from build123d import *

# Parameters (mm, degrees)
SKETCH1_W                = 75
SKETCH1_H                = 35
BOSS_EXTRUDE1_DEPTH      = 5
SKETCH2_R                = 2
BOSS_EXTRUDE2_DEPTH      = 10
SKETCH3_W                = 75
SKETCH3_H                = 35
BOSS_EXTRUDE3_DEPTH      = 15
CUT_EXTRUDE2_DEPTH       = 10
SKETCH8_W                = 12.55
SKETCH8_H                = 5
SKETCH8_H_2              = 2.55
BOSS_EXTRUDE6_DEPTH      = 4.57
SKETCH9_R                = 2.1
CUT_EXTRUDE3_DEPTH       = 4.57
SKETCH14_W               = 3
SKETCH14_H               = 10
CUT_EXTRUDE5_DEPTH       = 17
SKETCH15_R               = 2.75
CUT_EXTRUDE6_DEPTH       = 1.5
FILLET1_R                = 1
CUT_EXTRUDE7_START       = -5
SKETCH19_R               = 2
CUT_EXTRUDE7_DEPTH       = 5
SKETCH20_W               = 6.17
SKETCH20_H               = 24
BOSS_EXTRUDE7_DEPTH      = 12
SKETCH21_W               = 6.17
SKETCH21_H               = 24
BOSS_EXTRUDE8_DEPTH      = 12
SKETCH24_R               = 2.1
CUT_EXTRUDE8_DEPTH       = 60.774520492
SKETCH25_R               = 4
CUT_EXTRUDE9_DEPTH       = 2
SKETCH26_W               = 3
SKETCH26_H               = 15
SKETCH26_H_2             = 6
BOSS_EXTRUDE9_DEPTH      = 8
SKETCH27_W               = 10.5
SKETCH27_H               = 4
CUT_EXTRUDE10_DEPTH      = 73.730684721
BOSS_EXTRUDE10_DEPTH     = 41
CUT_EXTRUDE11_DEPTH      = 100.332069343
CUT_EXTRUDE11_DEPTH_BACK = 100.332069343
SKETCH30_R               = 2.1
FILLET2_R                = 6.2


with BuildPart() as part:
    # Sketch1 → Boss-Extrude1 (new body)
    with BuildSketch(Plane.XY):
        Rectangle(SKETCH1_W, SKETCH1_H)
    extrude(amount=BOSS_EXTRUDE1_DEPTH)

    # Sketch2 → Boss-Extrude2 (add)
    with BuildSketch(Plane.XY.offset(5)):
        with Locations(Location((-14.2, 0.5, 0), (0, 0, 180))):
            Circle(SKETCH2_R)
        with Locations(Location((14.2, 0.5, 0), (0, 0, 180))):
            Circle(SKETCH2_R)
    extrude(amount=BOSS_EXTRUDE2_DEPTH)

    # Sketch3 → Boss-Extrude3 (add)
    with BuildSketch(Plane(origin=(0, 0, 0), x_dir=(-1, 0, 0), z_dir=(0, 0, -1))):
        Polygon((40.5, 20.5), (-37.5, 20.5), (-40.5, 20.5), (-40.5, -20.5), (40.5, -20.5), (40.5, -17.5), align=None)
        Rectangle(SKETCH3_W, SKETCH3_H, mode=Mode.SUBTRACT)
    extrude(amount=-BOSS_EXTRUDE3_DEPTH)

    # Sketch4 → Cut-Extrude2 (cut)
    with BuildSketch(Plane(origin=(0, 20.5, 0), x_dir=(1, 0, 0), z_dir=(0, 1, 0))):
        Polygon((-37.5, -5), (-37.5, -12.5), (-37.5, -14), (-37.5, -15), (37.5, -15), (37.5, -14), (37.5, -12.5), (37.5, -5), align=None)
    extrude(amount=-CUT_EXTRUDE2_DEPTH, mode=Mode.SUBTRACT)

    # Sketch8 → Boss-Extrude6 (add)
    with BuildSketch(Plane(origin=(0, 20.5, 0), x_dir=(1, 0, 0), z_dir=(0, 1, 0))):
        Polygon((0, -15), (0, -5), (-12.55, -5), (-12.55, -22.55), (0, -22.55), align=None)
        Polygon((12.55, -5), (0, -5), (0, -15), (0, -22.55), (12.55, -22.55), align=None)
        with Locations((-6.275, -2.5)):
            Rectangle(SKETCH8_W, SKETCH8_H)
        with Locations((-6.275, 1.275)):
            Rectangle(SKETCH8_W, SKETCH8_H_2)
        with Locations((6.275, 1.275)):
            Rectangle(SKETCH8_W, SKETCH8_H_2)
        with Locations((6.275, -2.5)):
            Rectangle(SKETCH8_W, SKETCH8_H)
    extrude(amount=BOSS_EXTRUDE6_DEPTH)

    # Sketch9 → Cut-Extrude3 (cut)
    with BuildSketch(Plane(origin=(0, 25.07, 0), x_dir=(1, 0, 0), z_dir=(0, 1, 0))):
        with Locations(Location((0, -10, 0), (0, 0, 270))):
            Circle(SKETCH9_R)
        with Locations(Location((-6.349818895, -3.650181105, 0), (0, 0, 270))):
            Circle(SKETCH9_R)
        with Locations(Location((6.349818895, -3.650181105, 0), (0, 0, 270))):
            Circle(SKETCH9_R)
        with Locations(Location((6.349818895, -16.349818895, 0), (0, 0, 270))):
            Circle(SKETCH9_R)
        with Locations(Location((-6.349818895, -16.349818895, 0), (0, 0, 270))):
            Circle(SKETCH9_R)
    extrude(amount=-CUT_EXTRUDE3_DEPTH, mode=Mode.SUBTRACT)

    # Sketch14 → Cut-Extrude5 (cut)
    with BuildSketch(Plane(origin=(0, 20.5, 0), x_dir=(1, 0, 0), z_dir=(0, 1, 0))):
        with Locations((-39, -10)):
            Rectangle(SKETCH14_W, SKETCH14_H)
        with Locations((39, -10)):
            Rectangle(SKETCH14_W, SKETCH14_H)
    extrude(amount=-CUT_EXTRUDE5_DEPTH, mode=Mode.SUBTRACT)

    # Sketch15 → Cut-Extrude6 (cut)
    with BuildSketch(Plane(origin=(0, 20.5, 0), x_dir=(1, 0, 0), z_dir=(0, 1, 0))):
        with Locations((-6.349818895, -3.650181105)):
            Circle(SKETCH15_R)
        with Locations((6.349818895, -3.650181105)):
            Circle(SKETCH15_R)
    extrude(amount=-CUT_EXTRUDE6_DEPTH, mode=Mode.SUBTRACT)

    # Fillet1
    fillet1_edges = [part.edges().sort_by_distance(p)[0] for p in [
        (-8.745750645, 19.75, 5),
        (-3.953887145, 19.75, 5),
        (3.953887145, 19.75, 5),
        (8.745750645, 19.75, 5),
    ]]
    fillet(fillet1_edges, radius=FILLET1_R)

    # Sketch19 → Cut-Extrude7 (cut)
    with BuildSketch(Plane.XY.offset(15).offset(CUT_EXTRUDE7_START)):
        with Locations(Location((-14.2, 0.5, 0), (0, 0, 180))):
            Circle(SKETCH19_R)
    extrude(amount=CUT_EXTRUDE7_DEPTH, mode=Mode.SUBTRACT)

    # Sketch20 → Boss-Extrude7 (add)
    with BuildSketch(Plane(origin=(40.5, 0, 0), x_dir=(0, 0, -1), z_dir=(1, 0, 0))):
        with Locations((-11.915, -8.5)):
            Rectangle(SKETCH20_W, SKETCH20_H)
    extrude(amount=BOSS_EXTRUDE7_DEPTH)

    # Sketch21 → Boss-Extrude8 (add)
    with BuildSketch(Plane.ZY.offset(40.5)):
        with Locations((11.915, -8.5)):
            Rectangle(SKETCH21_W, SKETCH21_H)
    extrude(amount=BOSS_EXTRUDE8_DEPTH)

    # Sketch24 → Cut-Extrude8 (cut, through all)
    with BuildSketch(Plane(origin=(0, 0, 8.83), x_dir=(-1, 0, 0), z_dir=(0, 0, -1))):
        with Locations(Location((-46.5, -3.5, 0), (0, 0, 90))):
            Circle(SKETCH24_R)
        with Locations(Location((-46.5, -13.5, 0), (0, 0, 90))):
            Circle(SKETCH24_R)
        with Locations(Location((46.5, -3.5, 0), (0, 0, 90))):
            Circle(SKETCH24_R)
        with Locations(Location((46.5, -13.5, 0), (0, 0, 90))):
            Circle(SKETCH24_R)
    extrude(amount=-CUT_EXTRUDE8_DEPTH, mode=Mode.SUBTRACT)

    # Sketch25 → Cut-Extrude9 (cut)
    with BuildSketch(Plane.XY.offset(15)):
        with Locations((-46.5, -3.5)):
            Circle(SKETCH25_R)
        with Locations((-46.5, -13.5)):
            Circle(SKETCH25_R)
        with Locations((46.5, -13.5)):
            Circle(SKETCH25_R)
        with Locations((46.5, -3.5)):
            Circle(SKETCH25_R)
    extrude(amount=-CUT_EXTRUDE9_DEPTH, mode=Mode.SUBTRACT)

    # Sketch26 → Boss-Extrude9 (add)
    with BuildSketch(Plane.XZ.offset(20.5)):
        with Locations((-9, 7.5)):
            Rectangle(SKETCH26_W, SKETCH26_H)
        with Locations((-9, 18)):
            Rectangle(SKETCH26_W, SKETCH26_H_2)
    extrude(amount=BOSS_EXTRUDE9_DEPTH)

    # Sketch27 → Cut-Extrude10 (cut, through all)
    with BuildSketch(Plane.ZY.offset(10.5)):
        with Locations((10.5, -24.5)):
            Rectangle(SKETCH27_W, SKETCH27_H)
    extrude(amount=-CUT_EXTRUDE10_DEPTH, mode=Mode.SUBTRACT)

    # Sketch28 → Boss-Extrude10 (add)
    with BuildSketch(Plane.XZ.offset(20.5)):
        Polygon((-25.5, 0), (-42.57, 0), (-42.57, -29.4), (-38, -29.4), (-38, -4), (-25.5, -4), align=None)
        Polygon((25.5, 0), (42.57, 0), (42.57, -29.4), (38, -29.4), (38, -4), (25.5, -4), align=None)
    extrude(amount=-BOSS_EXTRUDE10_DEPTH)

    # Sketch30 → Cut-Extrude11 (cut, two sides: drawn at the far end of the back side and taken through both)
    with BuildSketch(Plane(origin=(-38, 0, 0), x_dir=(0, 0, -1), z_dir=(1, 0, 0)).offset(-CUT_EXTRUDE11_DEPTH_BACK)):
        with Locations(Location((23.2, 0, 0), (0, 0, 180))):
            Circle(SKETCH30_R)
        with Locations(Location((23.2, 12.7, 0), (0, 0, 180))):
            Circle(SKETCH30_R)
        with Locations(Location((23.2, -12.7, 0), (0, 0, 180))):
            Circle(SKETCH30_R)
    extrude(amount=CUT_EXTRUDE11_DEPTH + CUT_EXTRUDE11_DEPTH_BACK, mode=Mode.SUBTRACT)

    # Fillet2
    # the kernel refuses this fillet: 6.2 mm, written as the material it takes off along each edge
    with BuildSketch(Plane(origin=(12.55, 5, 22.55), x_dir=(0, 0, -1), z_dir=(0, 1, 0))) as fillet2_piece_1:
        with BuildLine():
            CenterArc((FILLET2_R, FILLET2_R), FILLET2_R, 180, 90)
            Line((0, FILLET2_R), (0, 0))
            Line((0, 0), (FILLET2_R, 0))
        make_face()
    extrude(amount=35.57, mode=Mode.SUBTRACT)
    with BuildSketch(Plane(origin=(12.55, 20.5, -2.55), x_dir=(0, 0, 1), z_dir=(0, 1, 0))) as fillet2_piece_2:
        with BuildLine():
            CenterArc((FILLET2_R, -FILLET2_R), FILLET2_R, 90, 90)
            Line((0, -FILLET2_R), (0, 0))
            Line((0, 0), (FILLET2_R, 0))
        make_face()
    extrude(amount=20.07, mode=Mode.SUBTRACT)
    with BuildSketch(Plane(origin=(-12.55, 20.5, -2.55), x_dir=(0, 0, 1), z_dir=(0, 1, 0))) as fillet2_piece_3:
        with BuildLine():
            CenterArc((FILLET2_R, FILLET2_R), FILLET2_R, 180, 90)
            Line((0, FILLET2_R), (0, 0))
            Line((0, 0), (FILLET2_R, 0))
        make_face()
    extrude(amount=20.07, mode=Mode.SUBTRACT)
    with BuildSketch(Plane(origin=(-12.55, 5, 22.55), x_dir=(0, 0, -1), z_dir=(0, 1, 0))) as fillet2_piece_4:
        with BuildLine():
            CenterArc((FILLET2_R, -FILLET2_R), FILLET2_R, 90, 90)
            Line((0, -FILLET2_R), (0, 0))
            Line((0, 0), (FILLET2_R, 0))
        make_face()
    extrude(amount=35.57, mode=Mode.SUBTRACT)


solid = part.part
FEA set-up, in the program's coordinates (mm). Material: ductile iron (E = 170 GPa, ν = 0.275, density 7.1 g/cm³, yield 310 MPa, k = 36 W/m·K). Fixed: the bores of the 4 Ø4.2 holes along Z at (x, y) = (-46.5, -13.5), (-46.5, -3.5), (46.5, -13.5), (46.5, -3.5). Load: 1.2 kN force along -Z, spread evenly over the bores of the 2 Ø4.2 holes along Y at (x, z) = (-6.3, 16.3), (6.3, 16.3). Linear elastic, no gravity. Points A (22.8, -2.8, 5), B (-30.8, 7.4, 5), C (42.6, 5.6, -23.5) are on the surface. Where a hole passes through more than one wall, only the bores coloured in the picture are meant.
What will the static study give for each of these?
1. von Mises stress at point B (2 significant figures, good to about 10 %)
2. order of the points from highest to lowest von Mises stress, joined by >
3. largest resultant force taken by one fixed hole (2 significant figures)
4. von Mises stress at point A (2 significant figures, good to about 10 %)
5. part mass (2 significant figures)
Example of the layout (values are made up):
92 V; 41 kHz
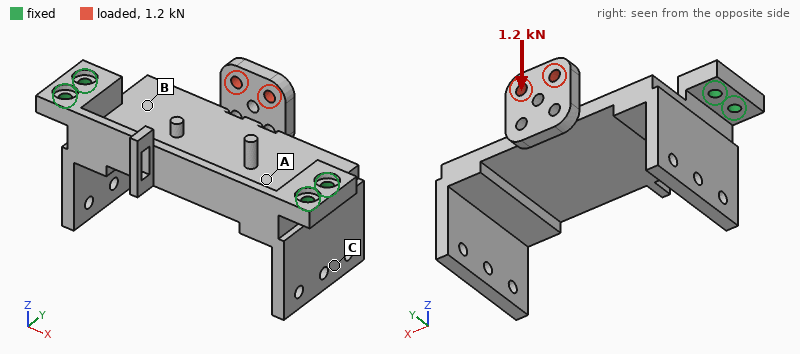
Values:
49 MPa; B > A > C; 1.8 kN; 33 MPa; 290 g
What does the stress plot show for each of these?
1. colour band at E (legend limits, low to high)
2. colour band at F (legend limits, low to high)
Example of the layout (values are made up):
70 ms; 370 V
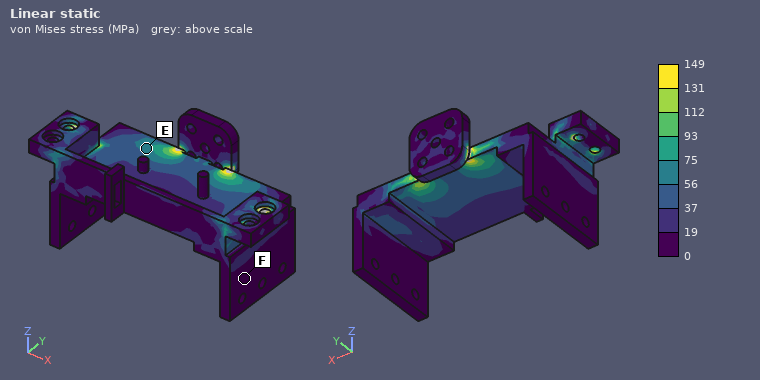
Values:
56 to 75 MPa; 0 to 19 MPa
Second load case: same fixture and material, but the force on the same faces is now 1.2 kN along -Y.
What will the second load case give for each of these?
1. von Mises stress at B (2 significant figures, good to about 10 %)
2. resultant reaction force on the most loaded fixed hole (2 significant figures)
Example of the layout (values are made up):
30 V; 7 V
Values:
32 MPa; 410 N
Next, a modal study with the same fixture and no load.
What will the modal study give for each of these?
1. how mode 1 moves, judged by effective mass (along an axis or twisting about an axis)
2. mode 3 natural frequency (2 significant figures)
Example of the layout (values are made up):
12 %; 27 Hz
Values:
along Z; 3000 Hz
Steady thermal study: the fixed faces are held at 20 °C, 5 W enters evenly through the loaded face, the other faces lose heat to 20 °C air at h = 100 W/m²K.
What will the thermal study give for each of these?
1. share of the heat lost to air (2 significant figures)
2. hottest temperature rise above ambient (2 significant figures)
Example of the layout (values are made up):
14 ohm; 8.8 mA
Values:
92 %; 24 K
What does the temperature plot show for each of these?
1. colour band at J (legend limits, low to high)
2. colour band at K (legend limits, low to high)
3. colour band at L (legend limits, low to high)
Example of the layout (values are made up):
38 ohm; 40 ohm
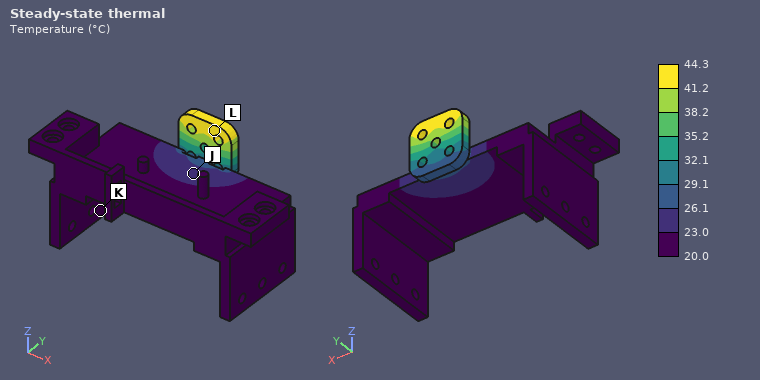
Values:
23.0 to 26.1 °C; 20.0 to 23.0 °C; 41.2 to 44.3 °C
